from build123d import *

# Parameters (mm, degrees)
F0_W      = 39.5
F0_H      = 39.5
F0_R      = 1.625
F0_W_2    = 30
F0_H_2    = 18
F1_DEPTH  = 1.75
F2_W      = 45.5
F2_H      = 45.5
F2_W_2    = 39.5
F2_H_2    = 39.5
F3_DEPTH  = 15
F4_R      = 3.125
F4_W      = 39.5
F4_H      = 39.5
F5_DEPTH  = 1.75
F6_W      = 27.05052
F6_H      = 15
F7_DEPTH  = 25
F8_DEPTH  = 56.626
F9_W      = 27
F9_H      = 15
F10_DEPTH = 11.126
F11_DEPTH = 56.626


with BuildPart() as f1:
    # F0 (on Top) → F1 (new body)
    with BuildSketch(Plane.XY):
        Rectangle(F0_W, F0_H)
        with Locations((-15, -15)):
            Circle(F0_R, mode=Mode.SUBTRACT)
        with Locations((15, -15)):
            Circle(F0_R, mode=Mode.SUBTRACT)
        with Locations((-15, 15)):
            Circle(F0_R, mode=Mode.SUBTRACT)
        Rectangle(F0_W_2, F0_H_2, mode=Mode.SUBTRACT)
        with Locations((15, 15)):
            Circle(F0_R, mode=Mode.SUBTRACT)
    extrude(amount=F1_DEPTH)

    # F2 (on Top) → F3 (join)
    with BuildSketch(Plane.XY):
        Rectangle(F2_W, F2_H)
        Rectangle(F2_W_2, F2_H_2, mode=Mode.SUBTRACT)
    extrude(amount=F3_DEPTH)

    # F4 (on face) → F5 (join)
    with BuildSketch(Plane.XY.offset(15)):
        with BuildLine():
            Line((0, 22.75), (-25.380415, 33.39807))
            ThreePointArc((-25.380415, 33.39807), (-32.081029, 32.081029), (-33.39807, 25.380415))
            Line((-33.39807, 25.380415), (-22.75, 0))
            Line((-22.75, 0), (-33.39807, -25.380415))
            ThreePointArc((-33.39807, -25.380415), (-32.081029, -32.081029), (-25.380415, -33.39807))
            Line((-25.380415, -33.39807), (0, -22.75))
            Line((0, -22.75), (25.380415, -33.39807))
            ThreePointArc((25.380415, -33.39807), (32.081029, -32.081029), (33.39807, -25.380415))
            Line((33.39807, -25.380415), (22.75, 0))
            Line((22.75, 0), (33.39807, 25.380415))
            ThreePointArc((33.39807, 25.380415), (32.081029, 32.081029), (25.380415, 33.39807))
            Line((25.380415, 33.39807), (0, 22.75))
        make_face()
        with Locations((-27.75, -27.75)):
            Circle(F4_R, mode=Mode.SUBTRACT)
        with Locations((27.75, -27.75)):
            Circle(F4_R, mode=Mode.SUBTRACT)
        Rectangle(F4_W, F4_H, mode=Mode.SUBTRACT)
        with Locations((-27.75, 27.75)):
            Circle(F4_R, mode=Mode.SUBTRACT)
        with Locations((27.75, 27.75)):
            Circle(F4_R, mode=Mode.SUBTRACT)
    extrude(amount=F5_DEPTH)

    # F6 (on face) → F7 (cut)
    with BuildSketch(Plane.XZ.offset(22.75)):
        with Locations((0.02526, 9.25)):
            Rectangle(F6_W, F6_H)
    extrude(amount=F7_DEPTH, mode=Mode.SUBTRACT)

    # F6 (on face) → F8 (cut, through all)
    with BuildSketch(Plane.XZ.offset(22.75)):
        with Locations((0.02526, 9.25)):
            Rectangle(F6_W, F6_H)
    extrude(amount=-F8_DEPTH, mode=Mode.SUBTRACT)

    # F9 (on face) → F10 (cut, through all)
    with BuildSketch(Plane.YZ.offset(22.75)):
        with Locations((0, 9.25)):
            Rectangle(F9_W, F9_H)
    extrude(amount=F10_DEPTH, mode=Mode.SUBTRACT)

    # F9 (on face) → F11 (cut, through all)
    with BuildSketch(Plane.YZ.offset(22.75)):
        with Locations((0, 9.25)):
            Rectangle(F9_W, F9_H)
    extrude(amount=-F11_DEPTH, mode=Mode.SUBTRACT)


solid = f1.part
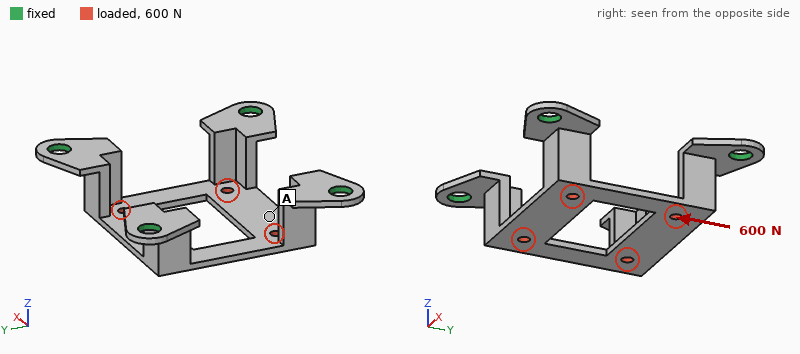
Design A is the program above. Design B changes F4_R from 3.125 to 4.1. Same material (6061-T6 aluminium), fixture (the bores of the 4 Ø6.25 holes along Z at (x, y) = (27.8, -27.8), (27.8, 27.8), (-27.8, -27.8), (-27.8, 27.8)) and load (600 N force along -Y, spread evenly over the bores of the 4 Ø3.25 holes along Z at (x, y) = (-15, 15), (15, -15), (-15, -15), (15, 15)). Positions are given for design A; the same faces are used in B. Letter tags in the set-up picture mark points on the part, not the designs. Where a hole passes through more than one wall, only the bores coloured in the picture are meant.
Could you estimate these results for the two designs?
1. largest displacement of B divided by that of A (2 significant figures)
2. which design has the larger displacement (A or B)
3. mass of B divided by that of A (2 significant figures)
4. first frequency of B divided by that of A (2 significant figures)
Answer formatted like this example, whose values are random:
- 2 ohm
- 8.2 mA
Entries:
- 0.90
- A
- 0.98
- 1.1
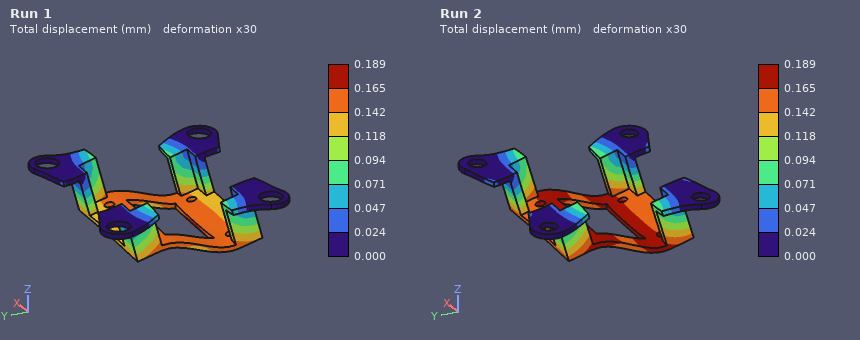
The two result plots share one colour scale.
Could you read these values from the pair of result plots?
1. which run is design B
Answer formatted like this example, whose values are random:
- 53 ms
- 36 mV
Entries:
- Run 1
